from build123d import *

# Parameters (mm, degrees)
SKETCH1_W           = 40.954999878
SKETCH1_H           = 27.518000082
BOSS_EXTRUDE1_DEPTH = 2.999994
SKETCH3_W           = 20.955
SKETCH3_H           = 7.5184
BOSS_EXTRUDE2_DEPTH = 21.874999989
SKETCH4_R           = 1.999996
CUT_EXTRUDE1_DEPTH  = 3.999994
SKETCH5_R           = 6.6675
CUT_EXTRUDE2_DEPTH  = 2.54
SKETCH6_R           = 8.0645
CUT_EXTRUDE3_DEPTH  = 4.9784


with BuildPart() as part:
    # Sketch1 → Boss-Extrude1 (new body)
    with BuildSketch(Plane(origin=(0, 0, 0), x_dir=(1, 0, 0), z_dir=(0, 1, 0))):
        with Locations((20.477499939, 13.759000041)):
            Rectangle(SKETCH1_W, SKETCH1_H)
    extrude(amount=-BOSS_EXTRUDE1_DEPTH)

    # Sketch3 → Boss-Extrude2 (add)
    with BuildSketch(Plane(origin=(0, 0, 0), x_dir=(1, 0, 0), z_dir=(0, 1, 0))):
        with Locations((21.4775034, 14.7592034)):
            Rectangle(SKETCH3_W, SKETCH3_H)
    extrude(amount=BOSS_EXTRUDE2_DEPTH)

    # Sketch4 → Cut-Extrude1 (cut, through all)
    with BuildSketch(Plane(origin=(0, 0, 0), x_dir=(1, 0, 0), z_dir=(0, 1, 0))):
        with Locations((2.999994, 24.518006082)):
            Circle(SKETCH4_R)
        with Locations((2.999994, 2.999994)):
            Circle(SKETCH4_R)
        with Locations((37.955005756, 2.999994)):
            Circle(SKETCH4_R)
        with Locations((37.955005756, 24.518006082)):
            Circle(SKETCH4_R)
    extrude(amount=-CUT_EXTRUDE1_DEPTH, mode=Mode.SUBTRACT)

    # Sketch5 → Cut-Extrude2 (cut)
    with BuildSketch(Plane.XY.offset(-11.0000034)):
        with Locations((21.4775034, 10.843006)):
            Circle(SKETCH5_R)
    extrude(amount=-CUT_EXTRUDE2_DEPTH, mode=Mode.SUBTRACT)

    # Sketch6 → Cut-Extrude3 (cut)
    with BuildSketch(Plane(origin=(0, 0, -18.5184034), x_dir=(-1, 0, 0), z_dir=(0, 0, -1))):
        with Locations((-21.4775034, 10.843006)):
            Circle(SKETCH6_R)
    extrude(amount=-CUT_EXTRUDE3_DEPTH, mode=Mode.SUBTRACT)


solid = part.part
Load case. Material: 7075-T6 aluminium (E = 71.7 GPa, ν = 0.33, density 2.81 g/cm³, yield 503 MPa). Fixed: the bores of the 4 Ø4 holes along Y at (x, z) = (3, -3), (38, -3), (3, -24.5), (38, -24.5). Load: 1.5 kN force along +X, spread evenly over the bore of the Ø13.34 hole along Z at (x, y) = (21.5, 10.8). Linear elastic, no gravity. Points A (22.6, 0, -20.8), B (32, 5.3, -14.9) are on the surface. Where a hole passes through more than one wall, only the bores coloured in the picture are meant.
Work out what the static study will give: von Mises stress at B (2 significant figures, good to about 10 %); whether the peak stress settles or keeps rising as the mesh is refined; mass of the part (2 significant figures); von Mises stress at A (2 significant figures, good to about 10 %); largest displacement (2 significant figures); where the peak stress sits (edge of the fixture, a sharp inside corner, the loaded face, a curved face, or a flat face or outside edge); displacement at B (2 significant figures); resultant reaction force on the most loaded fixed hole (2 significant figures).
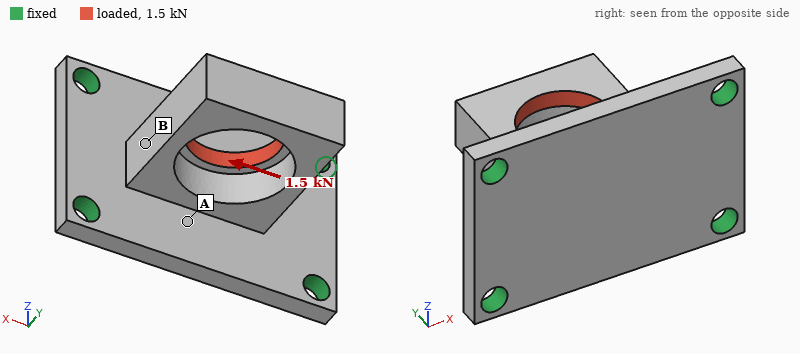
83 MPa
keeps rising
15 g
19 MPa
0.10 mm
edge of the fixture
0.031 mm
590 N
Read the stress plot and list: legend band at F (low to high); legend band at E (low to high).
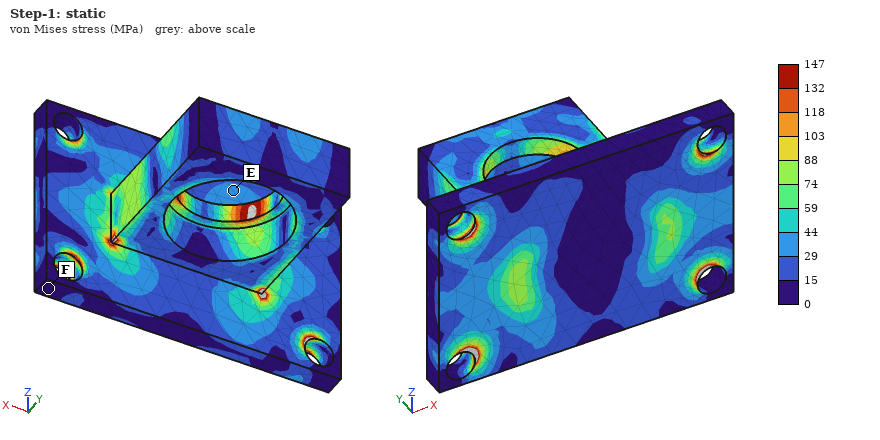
0 to 15 MPa
29 to 44 MPa
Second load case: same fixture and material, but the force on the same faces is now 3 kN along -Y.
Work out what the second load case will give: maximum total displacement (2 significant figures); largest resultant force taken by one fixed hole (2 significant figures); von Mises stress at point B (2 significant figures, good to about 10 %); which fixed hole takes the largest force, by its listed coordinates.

0.15 mm
960 N
65 MPa
(38, -3)
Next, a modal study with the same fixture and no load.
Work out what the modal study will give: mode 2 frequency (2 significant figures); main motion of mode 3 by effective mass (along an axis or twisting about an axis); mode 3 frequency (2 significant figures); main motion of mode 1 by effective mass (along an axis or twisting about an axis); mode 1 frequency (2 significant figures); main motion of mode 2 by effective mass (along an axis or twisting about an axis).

8600 Hz
along Y
11 kHz
along Z
5900 Hz
along X
